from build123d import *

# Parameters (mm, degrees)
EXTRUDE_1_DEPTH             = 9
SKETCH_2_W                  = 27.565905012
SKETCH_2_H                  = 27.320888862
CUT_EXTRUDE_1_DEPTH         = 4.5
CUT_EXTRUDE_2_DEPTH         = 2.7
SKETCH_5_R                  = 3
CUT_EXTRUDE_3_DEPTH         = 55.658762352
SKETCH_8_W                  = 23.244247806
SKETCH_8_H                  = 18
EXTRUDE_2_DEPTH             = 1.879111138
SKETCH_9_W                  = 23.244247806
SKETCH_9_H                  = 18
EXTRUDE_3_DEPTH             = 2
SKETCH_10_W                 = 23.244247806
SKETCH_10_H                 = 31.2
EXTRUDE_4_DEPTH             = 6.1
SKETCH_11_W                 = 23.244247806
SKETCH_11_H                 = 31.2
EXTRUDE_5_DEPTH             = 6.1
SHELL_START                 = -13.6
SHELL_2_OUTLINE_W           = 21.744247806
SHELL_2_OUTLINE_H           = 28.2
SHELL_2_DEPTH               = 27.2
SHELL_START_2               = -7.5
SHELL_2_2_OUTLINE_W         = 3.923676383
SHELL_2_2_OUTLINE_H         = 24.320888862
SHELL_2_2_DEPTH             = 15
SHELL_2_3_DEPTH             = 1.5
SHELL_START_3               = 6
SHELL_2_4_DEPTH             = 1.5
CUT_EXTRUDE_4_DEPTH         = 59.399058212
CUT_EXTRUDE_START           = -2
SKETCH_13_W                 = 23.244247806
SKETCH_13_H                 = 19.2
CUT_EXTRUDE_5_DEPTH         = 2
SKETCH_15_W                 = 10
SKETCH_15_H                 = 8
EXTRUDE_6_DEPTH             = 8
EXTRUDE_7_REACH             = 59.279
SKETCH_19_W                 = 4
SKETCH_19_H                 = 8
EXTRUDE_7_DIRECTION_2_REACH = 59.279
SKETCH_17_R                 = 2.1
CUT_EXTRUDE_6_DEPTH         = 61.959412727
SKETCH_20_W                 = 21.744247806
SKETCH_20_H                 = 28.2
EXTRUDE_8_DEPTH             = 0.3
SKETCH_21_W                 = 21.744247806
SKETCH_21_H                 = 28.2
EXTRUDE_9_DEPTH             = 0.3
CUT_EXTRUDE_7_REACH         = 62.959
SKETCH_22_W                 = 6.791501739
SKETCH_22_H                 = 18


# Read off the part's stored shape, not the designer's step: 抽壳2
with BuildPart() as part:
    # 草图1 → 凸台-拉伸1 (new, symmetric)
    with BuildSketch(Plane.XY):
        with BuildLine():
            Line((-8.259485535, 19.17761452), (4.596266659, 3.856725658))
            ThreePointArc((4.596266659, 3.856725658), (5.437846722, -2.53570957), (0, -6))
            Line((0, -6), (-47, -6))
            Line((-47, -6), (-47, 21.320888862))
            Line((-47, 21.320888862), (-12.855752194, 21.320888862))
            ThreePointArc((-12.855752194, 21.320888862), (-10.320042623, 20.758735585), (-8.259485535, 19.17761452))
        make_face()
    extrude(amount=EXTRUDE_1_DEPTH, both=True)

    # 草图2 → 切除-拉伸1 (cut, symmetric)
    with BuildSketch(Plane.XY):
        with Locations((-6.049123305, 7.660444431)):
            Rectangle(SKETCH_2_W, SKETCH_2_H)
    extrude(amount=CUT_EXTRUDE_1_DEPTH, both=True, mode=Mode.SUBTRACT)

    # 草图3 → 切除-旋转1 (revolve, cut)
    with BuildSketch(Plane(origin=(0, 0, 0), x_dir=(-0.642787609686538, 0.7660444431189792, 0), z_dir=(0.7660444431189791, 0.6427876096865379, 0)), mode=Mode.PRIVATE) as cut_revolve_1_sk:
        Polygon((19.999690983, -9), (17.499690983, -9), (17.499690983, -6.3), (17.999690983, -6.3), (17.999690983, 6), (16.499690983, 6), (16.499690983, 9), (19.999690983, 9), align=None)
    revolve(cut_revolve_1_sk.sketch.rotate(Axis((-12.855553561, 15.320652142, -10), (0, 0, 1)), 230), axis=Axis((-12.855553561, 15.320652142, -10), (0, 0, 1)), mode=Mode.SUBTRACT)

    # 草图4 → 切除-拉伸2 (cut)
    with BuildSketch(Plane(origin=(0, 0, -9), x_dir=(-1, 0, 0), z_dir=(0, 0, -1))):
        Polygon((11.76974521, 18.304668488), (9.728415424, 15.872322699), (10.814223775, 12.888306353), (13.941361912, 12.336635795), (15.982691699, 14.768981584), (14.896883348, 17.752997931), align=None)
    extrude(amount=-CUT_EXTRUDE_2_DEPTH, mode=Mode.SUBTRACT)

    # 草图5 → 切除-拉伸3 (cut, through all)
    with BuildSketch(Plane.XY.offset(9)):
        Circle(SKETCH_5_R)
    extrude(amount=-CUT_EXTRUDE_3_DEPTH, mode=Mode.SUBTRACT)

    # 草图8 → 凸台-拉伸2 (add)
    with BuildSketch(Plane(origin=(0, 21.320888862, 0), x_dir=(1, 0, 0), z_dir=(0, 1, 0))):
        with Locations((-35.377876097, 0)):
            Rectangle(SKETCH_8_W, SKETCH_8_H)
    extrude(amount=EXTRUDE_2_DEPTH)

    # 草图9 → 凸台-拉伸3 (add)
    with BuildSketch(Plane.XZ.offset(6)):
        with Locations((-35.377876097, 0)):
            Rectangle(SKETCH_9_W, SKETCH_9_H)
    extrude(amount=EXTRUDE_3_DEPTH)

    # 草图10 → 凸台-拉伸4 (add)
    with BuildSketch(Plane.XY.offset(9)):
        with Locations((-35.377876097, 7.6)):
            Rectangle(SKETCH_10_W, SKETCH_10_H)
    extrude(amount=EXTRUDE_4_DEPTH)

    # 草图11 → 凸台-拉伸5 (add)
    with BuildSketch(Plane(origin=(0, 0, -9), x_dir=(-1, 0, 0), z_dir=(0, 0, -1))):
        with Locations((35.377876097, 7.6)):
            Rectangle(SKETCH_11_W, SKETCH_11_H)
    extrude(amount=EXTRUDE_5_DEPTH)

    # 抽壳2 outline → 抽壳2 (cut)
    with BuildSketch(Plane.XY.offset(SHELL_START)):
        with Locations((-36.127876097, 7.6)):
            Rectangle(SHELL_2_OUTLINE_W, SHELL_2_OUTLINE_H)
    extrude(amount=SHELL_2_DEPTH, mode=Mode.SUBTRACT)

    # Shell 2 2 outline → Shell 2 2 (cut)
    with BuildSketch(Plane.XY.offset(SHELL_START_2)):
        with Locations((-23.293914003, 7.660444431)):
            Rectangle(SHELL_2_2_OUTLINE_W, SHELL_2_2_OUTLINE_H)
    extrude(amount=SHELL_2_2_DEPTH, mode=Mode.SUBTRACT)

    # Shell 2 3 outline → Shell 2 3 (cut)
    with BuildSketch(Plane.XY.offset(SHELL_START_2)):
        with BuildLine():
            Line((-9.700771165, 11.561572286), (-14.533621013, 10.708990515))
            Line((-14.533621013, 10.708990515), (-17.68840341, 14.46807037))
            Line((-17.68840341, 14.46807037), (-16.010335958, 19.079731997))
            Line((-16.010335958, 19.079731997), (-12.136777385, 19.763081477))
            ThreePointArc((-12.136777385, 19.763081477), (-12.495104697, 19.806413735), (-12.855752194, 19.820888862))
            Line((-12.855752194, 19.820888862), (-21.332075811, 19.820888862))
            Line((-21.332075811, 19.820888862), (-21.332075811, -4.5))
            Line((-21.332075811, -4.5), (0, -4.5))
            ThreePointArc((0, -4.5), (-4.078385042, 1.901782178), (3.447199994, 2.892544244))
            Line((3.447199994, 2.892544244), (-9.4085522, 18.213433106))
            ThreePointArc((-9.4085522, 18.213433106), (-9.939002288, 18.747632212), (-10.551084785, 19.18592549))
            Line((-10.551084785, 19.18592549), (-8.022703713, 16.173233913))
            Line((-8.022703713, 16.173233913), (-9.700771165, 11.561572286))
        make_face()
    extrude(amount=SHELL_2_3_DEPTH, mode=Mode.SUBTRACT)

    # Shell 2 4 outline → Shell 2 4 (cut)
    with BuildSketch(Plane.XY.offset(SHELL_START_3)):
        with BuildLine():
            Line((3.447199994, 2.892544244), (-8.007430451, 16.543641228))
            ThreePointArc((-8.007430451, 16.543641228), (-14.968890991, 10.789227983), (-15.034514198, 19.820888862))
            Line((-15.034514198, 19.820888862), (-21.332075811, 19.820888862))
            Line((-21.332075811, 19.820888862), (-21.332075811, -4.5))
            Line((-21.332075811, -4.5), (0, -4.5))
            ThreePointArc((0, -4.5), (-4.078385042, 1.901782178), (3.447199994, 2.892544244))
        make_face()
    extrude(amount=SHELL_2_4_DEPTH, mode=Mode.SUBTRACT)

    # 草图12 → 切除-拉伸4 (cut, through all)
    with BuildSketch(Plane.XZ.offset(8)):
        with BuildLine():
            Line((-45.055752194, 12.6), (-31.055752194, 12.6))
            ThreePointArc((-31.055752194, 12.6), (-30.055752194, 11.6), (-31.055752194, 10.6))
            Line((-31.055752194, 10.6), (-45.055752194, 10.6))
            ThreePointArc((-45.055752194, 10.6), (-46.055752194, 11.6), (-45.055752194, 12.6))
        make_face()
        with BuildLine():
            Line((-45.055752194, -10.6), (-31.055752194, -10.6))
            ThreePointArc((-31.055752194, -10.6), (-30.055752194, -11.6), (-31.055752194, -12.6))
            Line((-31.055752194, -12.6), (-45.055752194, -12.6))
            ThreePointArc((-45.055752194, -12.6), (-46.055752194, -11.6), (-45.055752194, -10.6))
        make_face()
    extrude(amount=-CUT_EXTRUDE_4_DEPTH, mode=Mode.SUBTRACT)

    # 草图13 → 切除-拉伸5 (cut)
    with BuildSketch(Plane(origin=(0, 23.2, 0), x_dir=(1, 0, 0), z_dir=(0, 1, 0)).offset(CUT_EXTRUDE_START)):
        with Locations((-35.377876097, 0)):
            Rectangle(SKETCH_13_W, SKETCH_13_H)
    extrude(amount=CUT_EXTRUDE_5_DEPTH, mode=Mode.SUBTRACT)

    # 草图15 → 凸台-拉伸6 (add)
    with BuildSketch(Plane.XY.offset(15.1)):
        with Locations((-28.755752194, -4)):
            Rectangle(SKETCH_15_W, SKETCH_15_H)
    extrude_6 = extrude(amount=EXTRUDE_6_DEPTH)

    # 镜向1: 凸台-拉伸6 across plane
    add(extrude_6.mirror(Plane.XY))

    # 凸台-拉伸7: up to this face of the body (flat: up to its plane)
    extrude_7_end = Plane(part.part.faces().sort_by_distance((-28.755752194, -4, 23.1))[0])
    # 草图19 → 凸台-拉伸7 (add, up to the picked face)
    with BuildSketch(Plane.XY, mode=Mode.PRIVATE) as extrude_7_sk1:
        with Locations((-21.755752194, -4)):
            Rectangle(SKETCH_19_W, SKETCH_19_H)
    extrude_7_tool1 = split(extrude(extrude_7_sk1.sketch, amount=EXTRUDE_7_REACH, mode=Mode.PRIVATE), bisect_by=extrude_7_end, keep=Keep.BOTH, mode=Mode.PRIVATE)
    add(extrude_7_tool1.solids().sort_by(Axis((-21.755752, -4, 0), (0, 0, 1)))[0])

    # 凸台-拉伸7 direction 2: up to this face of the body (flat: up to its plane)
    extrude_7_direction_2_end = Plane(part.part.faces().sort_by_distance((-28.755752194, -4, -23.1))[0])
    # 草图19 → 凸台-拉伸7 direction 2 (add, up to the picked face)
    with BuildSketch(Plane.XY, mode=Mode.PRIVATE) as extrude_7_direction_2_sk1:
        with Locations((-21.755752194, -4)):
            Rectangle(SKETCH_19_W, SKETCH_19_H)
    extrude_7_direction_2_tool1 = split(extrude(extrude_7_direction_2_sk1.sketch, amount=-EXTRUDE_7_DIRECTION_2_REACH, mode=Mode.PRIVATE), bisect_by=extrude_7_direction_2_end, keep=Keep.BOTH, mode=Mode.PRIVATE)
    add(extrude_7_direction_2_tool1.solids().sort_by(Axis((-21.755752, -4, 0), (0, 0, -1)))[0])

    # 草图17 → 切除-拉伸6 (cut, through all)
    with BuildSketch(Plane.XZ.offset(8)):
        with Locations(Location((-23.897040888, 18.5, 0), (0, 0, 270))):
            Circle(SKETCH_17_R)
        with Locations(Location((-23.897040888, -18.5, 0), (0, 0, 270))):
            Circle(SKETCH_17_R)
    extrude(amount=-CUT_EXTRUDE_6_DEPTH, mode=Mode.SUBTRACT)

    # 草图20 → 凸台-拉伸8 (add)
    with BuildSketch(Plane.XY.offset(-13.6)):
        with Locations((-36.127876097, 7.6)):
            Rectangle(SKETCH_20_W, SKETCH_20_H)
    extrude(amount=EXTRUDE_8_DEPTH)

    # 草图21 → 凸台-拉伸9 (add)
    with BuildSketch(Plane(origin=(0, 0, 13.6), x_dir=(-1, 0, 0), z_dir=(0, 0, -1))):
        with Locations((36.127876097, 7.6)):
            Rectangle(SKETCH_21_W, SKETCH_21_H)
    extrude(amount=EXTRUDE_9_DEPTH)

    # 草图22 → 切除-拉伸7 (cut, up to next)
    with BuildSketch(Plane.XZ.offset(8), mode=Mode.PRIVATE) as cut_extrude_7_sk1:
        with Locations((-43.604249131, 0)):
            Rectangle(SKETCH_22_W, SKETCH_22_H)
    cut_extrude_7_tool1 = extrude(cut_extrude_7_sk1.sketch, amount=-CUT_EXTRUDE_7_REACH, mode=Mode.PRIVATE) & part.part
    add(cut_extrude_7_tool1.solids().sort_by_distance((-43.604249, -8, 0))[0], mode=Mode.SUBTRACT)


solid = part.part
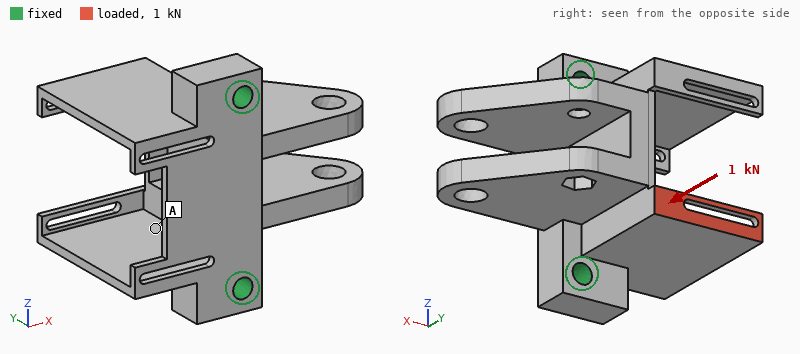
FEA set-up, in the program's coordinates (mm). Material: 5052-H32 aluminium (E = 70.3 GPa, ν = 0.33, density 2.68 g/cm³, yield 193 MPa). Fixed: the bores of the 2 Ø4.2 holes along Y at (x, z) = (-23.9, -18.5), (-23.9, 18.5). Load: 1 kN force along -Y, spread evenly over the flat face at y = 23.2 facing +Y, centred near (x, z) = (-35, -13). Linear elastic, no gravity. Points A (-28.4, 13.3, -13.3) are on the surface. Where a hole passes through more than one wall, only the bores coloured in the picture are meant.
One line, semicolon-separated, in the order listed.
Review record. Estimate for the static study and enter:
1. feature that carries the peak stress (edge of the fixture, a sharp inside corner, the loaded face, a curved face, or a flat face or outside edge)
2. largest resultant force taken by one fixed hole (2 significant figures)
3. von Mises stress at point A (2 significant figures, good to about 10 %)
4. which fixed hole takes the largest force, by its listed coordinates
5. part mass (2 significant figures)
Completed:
a curved face; 950 N; 36 MPa; (-23.9, -18.5); 29 g
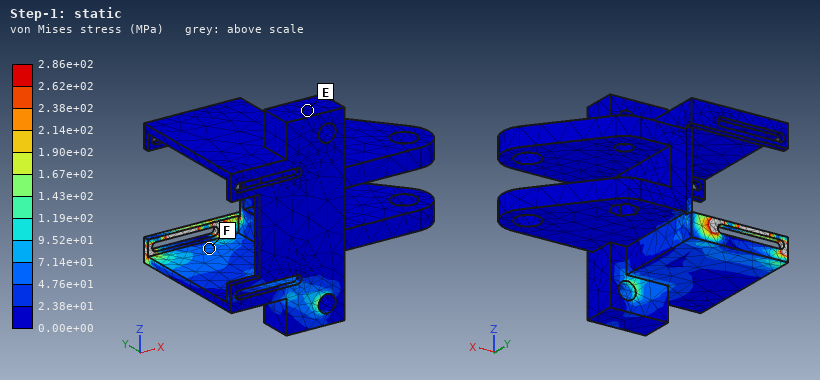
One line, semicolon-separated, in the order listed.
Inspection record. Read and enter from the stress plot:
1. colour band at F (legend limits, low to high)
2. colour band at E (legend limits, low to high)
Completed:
4.76e+01 to 7.14e+01 MPa; 0.00e+00 to 2.38e+01 MPa
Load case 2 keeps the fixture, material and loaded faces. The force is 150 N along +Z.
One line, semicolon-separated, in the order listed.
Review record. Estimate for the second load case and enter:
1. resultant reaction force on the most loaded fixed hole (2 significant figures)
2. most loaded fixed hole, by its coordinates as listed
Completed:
170 N; (-23.9, -18.5)
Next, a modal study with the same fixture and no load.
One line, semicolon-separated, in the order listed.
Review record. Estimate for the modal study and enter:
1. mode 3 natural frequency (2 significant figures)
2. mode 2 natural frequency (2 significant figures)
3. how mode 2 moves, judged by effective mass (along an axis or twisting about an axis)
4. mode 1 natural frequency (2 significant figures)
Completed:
4400 Hz; 3800 Hz; along Z; 3300 Hz
